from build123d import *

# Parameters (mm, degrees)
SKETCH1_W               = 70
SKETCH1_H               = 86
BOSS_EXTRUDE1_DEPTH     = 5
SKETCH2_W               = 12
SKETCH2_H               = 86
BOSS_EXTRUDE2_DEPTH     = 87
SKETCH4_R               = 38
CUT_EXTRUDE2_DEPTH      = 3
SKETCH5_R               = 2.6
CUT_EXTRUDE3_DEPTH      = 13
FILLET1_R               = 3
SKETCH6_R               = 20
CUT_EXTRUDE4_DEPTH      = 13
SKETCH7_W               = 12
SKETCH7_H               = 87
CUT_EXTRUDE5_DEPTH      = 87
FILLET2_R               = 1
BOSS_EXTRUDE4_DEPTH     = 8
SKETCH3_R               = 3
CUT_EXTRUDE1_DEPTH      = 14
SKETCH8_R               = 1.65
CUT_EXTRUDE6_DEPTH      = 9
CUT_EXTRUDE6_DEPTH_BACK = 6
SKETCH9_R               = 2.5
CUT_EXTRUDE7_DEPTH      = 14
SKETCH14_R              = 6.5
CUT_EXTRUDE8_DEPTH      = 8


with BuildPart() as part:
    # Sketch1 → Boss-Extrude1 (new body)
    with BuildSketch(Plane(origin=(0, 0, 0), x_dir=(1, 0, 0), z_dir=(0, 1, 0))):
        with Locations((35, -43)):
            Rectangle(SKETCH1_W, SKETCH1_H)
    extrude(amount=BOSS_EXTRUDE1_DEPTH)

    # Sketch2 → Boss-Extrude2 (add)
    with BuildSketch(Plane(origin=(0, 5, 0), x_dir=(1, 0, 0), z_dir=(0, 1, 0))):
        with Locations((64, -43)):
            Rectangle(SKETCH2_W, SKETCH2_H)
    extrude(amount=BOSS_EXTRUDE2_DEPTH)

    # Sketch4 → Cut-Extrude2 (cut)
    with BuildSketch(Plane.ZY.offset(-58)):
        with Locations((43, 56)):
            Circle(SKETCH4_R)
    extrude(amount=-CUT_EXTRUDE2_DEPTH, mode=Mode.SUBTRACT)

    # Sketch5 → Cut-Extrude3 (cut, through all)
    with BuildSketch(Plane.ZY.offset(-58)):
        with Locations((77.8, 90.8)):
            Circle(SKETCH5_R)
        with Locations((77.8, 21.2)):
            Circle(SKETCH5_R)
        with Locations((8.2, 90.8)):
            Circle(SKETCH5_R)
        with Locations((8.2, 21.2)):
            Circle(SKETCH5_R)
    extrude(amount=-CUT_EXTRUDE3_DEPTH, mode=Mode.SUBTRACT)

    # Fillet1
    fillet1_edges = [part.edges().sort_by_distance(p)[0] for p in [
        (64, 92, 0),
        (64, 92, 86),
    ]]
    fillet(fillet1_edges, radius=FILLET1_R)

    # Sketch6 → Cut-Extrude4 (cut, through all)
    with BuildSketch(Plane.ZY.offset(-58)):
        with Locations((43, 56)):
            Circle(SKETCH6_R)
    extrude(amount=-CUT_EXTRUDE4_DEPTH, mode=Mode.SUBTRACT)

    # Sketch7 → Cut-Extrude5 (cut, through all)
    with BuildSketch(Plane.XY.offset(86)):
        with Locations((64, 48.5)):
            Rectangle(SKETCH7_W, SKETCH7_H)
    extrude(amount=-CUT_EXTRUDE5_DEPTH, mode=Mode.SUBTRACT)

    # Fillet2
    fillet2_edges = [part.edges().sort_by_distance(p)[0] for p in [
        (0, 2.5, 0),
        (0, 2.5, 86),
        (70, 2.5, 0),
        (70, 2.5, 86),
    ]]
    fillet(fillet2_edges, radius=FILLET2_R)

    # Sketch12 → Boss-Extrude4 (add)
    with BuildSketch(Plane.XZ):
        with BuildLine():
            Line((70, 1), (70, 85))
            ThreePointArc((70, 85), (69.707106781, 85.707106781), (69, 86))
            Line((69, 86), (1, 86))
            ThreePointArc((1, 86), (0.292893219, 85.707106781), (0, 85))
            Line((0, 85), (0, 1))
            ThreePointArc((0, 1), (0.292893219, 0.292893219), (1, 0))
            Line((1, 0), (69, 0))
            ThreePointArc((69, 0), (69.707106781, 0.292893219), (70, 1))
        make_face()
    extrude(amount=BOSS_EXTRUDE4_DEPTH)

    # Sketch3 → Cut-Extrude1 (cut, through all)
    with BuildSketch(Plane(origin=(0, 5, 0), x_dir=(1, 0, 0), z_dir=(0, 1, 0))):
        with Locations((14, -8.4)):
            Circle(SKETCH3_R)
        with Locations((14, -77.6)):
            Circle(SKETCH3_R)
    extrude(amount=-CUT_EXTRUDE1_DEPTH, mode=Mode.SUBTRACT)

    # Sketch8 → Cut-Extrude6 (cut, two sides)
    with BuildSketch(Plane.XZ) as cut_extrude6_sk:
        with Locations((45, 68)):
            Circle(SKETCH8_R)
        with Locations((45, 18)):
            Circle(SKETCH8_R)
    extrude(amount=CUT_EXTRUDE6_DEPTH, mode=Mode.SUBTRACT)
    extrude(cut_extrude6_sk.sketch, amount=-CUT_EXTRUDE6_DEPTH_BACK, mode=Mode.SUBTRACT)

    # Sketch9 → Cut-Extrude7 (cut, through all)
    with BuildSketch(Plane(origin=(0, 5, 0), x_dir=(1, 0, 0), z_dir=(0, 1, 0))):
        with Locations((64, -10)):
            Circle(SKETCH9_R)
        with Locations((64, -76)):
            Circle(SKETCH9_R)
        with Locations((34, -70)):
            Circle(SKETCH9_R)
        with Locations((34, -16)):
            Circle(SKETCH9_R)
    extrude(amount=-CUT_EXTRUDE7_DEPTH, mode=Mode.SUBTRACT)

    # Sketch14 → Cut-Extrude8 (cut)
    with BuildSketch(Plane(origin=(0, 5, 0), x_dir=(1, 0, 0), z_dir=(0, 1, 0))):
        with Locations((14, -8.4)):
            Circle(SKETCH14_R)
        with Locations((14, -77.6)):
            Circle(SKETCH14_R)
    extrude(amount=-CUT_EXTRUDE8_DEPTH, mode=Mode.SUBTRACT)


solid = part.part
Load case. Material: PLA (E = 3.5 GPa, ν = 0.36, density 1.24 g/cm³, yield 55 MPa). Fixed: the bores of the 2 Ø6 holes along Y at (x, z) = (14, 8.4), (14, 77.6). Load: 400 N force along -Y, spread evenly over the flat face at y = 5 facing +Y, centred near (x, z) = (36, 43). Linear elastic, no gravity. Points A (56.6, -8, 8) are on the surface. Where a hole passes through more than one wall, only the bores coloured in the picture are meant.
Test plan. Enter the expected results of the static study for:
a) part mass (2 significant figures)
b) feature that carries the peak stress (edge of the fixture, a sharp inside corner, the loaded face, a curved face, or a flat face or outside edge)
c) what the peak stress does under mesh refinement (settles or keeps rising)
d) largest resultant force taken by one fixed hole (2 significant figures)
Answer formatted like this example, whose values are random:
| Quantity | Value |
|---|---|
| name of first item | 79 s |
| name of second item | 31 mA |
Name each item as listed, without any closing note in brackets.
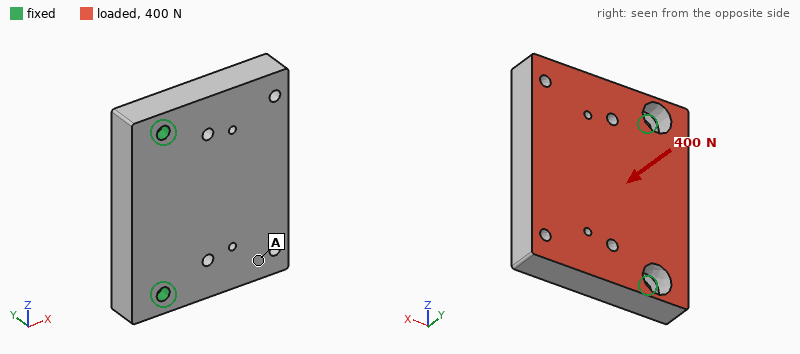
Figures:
| Quantity | Value |
|---|---|
| part mass | 93 g |
| feature that carries the peak stress | edge of the fixture |
| what the peak stress does under mesh refinement | keeps rising |
| largest resultant force taken by one fixed hole | 230 N |
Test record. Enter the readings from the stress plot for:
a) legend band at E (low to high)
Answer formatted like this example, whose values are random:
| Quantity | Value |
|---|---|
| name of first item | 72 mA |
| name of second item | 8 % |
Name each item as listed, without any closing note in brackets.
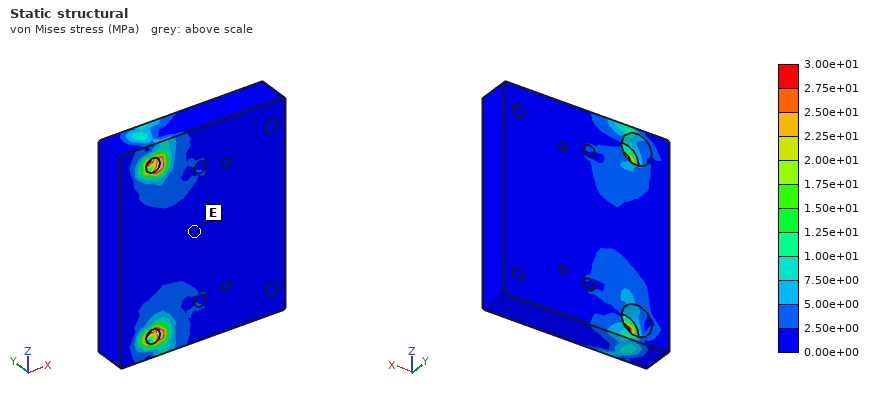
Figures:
| Quantity | Value |
|---|---|
| legend band at E | 0.00e+00 to 2.50e+00 MPa |
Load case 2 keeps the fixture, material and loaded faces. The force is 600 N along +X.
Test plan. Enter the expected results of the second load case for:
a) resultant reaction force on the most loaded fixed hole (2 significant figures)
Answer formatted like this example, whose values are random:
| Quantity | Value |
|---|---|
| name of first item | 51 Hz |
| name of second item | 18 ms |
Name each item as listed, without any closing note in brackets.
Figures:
| Quantity | Value |
|---|---|
| resultant reaction force on the most loaded fixed hole | 300 N |
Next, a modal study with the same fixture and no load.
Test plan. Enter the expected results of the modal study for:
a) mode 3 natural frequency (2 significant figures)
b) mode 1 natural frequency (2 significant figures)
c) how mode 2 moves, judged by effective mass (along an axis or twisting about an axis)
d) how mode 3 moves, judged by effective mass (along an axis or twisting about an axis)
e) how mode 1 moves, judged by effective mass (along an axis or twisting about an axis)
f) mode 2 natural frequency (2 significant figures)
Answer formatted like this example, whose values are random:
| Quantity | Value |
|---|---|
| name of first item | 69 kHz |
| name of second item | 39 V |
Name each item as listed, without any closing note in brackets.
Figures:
| Quantity | Value |
|---|---|
| mode 3 natural frequency | 2700 Hz |
| mode 1 natural frequency | 460 Hz |
| how mode 2 moves, judged by effective mass | twisting about X |
| how mode 3 moves, judged by effective mass | along Y |
| how mode 1 moves, judged by effective mass | along Y |
| mode 2 natural frequency | 1500 Hz |
